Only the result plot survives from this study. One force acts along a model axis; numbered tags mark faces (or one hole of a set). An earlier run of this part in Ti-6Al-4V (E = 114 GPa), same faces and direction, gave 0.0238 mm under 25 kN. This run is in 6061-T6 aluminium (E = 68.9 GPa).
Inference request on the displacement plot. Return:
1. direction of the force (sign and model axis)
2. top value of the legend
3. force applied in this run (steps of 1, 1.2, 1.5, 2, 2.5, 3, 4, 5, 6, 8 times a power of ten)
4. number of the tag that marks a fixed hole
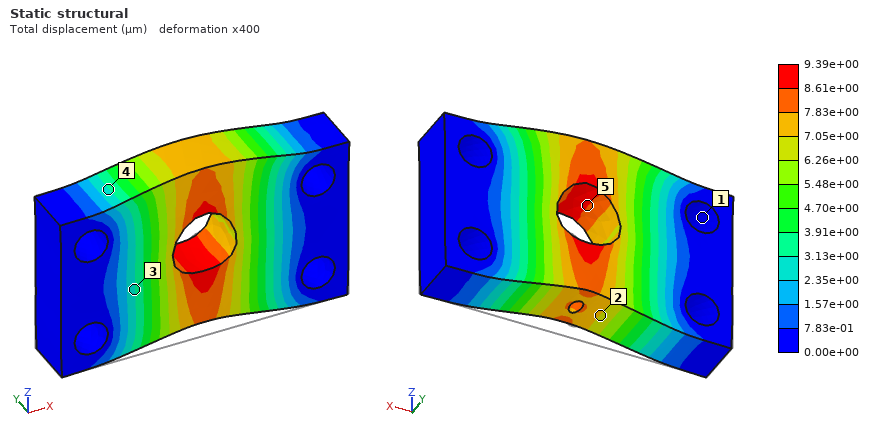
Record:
+Z
9.39e+00 µm
6 kN
1
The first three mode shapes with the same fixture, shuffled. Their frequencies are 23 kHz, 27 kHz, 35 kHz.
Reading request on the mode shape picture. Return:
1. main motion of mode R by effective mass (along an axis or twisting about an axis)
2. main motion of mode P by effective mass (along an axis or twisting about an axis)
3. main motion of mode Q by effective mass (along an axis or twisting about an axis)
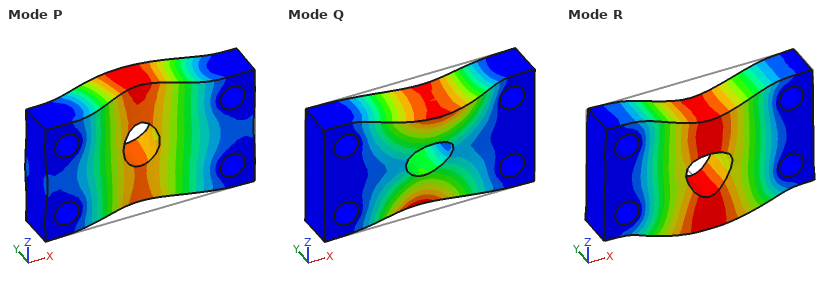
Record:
along Z
along Y
twisting about X
